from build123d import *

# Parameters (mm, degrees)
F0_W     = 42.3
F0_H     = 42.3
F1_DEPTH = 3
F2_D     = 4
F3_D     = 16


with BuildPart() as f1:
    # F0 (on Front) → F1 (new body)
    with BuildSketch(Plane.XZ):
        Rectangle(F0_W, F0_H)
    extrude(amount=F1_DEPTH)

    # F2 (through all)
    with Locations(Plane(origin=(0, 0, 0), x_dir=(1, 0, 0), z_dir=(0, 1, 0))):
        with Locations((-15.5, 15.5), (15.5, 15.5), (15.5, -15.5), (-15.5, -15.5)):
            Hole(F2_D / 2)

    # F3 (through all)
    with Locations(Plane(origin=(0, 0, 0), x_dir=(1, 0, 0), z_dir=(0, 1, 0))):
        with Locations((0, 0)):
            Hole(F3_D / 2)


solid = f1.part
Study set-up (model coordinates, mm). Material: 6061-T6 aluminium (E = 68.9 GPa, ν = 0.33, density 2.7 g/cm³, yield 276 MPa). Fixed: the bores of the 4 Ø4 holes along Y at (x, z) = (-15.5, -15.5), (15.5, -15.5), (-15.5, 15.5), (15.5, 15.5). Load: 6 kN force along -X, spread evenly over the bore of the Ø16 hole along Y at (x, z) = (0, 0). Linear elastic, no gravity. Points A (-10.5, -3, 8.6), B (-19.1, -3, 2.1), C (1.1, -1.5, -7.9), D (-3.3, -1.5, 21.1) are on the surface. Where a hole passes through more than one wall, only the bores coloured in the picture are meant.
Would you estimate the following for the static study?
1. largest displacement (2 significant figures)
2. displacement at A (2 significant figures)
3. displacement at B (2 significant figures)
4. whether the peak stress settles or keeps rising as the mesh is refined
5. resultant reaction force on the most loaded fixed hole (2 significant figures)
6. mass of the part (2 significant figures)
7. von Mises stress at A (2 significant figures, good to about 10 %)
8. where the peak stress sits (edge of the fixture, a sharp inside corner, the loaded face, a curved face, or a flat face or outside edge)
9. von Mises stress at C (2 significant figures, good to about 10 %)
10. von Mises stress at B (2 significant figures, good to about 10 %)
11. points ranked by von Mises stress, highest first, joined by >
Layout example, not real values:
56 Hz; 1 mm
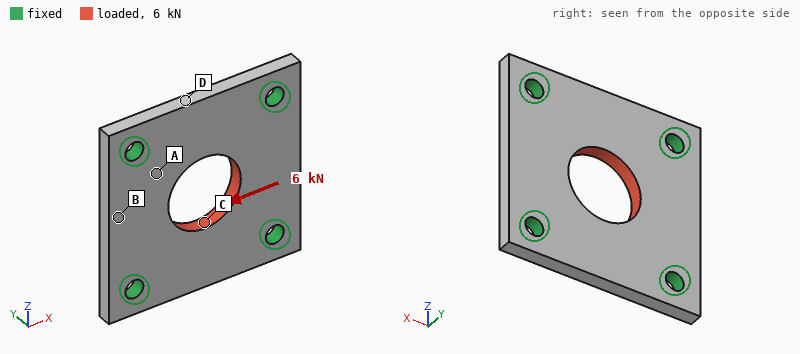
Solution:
16 µm; 8.3 µm; 12 µm; keeps rising; 1.6 kN; 12 g; 46 MPa; edge of the fixture; 69 MPa; 25 MPa; C > A > B > D
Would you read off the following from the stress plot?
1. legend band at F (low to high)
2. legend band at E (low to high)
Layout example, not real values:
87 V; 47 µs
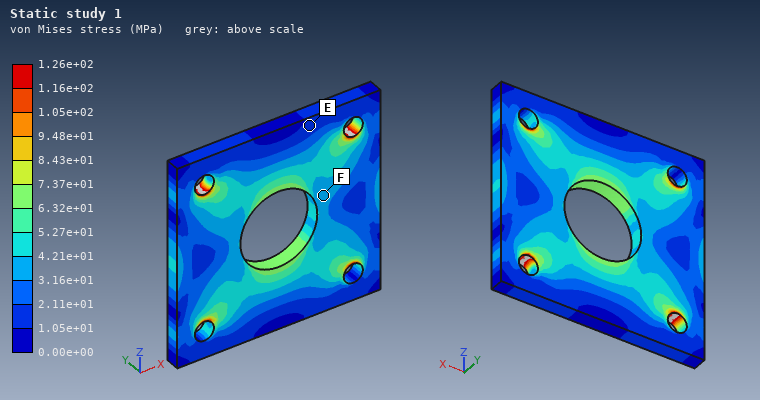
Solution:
3.16e+01 to 4.21e+01 MPa; 1.05e+01 to 2.11e+01 MPa
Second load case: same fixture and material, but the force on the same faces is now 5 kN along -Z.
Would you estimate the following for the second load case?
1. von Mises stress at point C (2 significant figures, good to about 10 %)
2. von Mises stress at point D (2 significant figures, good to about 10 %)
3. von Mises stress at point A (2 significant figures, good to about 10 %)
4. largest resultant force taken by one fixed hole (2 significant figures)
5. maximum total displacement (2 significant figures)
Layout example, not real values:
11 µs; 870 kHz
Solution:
37 MPa; 32 MPa; 38 MPa; 1.3 kN; 13 µm
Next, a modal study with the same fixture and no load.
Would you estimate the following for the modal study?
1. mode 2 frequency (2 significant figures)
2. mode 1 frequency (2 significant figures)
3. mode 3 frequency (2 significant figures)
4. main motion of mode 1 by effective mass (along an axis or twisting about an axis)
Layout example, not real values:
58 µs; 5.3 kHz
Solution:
18 kHz; 14 kHz; 18 kHz; along Y
